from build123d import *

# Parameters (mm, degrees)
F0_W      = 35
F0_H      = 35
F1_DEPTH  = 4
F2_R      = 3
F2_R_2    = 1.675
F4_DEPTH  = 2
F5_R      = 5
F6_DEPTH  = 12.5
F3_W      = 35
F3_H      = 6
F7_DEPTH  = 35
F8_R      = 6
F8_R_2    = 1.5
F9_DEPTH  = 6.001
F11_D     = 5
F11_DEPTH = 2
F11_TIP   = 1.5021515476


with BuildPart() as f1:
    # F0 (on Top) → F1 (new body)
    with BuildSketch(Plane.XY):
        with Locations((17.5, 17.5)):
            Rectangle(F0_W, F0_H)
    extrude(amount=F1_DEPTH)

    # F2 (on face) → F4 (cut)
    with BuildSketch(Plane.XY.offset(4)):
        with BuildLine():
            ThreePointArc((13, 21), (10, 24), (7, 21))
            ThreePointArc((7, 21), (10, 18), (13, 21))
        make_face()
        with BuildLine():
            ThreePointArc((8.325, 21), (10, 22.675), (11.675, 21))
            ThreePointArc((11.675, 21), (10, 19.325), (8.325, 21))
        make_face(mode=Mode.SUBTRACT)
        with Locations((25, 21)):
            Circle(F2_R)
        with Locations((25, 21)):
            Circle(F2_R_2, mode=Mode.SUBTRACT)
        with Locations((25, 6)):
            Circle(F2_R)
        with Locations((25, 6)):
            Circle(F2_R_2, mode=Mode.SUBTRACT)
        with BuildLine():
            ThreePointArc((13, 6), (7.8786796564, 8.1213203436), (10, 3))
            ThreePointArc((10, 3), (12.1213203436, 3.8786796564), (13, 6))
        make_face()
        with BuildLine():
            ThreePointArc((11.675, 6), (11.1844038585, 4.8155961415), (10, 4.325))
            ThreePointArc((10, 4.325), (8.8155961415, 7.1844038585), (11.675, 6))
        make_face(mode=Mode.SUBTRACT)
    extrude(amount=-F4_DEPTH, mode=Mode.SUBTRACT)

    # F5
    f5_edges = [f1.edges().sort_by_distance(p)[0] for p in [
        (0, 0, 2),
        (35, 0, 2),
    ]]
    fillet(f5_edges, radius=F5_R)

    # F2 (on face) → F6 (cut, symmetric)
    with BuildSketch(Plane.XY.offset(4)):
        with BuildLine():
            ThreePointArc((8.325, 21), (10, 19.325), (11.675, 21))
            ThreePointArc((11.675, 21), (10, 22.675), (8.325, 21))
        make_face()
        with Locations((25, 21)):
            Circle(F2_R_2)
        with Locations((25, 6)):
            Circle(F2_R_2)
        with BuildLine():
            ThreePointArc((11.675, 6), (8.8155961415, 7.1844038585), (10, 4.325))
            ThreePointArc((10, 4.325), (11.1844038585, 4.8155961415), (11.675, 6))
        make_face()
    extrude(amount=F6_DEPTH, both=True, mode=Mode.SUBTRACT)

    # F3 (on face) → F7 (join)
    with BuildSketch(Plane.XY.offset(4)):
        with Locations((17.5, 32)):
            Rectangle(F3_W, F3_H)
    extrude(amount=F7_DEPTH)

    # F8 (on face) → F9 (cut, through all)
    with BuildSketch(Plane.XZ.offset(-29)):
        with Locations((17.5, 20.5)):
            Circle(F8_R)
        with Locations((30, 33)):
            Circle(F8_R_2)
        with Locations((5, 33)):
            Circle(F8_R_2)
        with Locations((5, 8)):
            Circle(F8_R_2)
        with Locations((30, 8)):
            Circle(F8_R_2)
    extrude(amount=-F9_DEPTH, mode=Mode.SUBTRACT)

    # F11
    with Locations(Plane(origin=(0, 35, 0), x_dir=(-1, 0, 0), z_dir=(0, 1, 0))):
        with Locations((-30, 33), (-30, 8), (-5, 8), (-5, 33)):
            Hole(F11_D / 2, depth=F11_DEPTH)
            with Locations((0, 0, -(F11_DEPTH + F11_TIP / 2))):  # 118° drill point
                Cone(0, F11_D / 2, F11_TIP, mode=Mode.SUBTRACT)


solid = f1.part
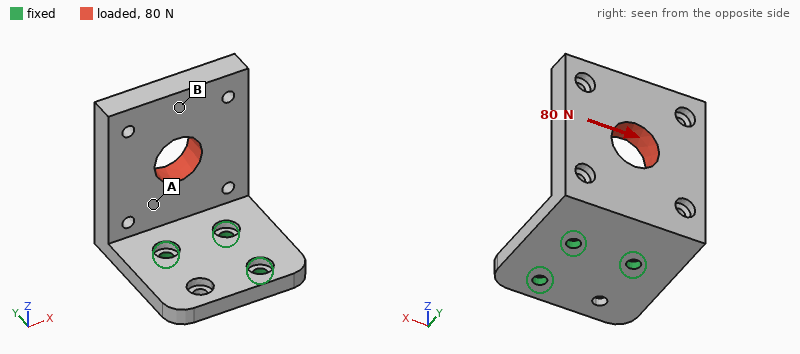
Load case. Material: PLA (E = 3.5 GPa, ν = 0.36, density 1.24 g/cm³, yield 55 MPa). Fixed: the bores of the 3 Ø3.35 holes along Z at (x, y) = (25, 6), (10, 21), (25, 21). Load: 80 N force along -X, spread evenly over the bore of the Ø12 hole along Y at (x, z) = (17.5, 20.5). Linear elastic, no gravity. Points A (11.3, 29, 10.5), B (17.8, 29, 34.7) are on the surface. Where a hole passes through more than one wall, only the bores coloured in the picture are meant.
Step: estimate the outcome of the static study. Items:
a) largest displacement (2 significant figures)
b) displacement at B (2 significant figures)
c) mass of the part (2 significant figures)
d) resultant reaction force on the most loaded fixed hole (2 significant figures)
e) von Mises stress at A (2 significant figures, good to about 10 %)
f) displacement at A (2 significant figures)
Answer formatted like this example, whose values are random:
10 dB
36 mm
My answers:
0.30 mm
0.24 mm
14 g
120 N
2.5 MPa
0.081 mm
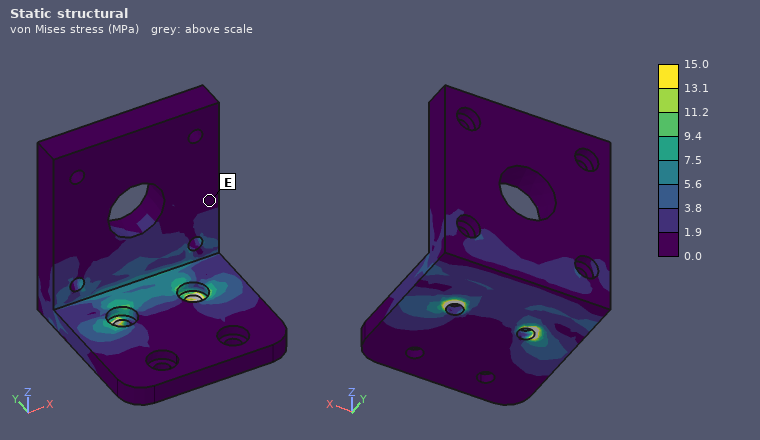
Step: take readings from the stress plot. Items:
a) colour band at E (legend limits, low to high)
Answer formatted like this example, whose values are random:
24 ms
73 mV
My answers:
0.0 to 1.9 MPa
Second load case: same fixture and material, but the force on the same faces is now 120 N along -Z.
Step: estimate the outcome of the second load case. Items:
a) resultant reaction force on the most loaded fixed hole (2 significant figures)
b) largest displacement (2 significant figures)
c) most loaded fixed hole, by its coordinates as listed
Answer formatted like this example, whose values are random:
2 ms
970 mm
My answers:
110 N
0.72 mm
(25, 21)
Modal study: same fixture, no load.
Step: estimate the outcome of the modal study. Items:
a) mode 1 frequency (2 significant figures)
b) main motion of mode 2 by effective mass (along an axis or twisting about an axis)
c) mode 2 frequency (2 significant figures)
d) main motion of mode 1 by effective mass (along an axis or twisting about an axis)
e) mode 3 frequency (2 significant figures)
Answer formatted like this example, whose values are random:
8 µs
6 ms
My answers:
480 Hz
along X
1000 Hz
along Y
2200 Hz
